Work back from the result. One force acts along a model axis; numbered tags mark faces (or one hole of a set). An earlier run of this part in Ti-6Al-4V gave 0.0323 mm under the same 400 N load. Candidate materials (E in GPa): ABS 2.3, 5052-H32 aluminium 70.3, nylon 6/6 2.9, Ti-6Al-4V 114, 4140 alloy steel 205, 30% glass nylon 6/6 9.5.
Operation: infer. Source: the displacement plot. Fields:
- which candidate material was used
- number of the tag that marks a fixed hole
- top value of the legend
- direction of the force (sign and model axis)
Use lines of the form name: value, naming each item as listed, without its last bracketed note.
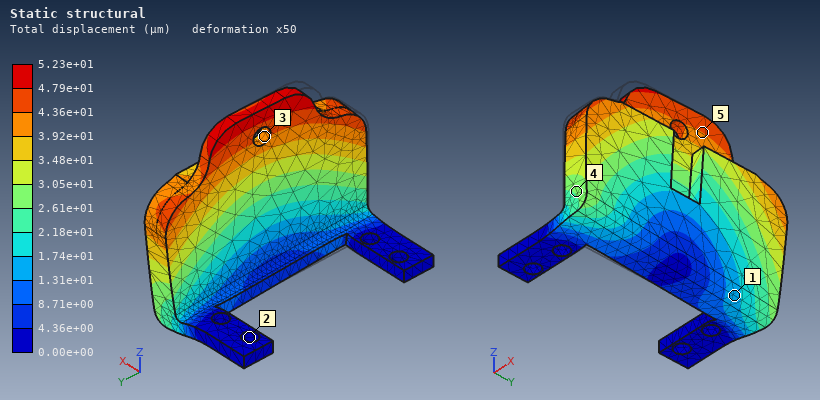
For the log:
which candidate material was used: 5052-H32 aluminium
number of the tag that marks a fixed hole: 2
top value of the legend: 5.23e+01 µm
direction of the force: +Y
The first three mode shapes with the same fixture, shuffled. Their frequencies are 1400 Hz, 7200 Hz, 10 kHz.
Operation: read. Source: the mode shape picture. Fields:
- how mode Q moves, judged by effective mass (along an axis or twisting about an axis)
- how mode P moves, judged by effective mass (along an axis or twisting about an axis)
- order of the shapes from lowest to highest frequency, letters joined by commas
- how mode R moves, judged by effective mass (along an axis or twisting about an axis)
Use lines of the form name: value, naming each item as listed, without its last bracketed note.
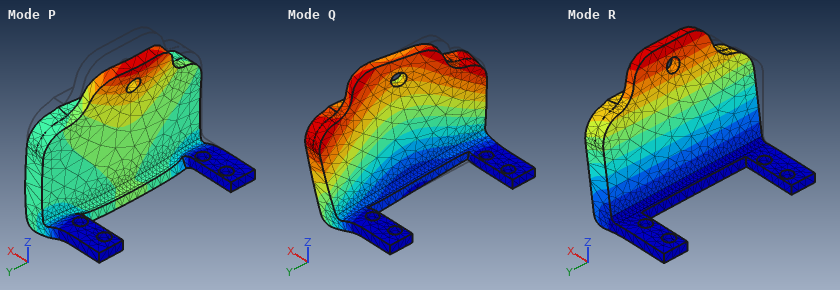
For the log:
how mode Q moves, judged by effective mass: along Y
how mode P moves, judged by effective mass: along Z
order of the shapes from lowest to highest frequency, letters joined by commas: R, Q, P
how mode R moves, judged by effective mass: along X
